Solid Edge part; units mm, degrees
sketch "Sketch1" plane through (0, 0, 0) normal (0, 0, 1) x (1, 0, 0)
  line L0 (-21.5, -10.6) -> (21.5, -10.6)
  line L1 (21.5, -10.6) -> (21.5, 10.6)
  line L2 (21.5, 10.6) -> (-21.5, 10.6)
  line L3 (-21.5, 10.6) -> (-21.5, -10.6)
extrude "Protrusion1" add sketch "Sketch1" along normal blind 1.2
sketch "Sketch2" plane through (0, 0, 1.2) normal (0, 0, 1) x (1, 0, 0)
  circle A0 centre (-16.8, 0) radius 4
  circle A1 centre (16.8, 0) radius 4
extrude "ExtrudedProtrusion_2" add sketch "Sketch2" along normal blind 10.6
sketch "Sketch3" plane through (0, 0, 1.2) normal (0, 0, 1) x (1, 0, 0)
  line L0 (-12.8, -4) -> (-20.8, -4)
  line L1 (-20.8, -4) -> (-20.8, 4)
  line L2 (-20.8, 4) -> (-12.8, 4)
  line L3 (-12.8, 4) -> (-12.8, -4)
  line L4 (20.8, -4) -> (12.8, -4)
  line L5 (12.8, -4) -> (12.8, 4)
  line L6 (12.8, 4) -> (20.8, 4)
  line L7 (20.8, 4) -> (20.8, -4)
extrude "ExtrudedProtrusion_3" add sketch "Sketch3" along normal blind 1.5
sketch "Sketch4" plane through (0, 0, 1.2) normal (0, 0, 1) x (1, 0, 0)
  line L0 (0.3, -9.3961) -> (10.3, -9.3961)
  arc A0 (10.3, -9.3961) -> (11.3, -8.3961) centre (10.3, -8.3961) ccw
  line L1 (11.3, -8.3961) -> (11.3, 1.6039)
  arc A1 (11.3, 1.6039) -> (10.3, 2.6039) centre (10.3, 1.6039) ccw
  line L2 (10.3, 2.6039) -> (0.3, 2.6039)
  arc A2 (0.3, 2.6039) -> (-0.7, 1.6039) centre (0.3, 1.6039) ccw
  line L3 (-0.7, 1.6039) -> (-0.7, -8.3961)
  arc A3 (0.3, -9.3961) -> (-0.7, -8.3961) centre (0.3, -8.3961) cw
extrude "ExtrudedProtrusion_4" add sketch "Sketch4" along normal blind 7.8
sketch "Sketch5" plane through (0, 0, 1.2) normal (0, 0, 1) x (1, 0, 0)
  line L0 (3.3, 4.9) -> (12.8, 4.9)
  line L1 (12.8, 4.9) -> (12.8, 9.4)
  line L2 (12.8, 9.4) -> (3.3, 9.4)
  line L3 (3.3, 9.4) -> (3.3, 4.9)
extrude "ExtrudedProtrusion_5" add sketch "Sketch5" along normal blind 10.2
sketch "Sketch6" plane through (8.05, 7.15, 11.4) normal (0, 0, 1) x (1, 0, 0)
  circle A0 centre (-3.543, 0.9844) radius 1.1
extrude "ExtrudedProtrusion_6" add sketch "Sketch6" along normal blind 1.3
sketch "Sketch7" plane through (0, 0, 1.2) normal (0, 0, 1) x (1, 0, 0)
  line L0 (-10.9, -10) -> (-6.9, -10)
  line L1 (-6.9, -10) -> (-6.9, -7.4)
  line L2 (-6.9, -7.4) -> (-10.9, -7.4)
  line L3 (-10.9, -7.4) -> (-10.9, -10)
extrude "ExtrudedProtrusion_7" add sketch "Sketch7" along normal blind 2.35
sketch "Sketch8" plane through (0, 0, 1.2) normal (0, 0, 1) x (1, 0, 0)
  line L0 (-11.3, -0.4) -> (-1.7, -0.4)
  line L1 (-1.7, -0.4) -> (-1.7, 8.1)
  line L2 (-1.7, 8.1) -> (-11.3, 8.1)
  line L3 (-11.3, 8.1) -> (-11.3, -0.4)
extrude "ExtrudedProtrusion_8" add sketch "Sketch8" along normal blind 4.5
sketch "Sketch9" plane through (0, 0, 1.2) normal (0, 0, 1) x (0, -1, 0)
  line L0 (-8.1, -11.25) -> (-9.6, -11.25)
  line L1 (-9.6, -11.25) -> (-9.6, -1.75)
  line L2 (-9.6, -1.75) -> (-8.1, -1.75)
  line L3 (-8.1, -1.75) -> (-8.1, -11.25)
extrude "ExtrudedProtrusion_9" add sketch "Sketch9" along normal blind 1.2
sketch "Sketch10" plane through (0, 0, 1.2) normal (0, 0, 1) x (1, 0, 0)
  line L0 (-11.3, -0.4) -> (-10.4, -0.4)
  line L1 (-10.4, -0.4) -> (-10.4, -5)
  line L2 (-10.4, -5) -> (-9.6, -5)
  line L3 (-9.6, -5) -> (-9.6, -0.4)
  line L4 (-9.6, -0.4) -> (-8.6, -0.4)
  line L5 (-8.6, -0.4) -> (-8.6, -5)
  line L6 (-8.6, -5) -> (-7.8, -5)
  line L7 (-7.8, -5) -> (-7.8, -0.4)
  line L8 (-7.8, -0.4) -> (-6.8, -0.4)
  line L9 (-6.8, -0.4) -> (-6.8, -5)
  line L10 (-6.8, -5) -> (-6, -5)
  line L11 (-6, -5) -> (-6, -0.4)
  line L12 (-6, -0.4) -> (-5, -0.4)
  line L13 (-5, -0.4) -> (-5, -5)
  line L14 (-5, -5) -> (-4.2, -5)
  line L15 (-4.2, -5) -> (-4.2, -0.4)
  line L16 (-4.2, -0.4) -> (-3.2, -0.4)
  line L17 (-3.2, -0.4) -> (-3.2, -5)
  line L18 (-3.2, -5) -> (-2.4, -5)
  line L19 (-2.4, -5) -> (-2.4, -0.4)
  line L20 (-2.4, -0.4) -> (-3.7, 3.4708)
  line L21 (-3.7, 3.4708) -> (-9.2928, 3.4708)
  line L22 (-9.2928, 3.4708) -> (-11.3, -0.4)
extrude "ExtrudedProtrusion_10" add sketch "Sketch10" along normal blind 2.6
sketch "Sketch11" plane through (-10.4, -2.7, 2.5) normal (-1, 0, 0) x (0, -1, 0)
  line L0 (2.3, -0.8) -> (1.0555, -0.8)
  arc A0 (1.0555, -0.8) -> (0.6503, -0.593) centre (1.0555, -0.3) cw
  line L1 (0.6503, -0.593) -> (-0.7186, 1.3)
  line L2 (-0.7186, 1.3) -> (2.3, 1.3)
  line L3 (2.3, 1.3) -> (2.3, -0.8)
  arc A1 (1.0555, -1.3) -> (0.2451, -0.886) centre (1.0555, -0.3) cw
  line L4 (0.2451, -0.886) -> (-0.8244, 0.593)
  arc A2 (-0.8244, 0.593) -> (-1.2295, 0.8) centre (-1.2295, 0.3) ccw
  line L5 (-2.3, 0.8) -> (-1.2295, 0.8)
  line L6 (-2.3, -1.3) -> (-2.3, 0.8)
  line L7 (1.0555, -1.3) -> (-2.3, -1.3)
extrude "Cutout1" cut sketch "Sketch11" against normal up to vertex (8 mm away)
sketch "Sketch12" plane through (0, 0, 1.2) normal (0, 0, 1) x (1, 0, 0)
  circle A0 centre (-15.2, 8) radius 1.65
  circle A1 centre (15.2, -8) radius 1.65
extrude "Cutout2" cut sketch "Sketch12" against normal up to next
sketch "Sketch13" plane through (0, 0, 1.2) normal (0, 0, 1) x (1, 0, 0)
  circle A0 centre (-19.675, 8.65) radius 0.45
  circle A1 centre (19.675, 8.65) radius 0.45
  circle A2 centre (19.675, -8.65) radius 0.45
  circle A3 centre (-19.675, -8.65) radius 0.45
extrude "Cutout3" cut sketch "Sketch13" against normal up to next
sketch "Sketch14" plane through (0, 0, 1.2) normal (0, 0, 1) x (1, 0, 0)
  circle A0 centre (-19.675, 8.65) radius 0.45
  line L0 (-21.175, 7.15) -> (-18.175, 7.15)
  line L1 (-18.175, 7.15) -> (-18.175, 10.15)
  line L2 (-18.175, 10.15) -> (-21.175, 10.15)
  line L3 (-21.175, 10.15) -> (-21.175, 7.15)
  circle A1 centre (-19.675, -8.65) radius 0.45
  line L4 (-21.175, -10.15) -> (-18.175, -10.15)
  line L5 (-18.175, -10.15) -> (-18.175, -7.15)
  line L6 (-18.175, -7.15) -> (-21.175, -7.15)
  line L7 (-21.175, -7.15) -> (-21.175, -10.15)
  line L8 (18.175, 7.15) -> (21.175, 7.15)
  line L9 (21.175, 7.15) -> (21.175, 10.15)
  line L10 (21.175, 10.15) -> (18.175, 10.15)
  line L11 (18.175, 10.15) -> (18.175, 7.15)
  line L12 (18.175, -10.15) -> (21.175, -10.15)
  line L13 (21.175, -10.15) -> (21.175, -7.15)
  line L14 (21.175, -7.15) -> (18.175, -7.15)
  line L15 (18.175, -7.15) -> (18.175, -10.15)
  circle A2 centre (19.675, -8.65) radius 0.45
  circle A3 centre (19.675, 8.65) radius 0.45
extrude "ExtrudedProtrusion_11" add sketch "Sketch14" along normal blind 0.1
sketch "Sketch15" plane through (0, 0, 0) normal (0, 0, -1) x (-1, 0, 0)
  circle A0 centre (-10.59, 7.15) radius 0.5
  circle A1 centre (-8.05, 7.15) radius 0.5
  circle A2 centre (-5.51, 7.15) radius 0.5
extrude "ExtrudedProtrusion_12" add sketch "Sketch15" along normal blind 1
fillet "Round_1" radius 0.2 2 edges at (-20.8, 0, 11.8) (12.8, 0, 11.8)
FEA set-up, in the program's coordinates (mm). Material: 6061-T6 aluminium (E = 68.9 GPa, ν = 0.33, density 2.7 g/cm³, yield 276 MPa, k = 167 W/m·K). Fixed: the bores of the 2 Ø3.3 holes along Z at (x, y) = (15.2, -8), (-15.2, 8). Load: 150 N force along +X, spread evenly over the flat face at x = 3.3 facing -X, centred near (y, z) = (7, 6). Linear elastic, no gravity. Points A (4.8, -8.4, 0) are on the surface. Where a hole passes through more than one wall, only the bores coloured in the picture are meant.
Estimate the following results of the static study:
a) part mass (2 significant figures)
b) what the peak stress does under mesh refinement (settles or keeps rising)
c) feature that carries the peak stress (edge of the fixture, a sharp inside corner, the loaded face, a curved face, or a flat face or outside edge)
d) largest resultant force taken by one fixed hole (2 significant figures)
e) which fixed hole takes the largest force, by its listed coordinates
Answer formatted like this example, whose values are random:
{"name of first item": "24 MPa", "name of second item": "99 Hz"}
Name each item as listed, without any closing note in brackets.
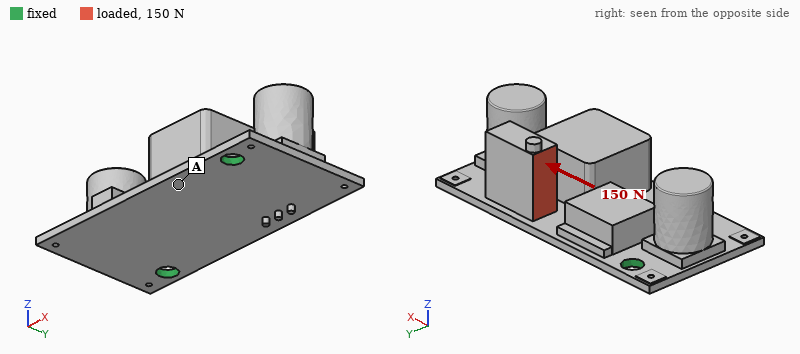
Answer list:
{"part mass": "11 g", "what the peak stress does under mesh refinement": "keeps rising", "feature that carries the peak stress": "edge of the fixture", "largest resultant force taken by one fixed hole": "91 N", "which fixed hole takes the largest force, by its listed coordinates": "(-15.2, 8)"}
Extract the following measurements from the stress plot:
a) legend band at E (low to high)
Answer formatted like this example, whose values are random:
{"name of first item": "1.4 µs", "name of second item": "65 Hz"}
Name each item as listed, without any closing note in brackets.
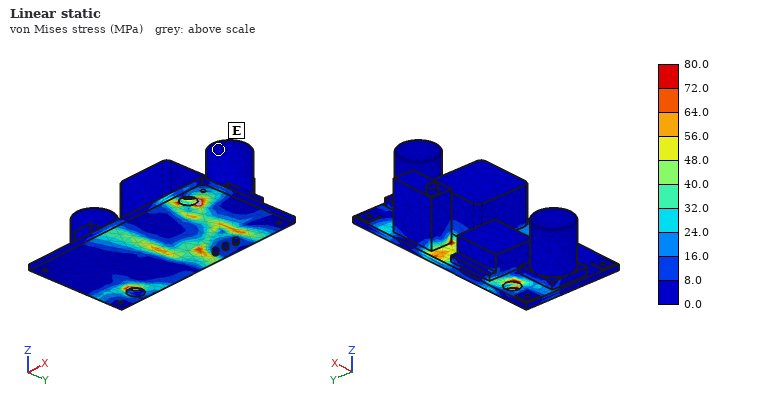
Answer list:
{"legend band at E": "0.0 to 8.0 MPa"}
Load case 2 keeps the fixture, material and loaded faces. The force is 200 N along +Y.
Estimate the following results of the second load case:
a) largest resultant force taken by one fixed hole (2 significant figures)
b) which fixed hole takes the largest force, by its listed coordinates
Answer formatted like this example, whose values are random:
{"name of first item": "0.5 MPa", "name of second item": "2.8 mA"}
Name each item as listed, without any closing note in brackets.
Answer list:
{"largest resultant force taken by one fixed hole": "120 N", "which fixed hole takes the largest force, by its listed coordinates": "(15.2, -8)"}
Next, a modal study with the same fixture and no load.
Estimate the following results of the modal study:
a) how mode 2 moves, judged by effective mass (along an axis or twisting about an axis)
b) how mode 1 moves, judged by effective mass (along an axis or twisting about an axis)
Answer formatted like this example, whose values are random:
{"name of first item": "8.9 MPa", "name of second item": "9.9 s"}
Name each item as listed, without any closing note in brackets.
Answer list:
{"how mode 2 moves, judged by effective mass": "along Z", "how mode 1 moves, judged by effective mass": "along Y"}
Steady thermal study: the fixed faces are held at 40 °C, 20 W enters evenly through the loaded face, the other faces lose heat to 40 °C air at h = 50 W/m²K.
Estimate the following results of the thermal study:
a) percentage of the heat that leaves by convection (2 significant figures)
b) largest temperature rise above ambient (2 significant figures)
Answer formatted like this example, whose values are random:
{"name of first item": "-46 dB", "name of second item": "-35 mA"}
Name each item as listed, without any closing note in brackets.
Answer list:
{"percentage of the heat that leaves by convection": "16 %", "largest temperature rise above ambient": "64 K"}
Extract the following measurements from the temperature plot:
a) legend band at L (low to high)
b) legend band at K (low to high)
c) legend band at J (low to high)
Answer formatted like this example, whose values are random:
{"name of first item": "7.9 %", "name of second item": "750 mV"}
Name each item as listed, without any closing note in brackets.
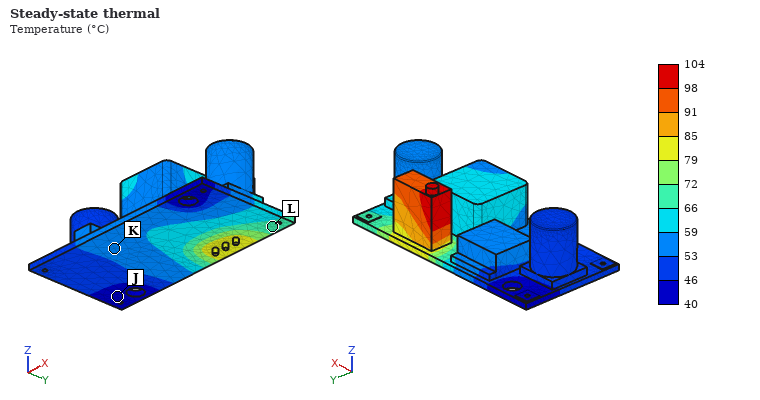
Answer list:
{"legend band at L": "66 to 72 °C", "legend band at K": "53 to 59 °C", "legend band at J": "40 to 46 °C"}
